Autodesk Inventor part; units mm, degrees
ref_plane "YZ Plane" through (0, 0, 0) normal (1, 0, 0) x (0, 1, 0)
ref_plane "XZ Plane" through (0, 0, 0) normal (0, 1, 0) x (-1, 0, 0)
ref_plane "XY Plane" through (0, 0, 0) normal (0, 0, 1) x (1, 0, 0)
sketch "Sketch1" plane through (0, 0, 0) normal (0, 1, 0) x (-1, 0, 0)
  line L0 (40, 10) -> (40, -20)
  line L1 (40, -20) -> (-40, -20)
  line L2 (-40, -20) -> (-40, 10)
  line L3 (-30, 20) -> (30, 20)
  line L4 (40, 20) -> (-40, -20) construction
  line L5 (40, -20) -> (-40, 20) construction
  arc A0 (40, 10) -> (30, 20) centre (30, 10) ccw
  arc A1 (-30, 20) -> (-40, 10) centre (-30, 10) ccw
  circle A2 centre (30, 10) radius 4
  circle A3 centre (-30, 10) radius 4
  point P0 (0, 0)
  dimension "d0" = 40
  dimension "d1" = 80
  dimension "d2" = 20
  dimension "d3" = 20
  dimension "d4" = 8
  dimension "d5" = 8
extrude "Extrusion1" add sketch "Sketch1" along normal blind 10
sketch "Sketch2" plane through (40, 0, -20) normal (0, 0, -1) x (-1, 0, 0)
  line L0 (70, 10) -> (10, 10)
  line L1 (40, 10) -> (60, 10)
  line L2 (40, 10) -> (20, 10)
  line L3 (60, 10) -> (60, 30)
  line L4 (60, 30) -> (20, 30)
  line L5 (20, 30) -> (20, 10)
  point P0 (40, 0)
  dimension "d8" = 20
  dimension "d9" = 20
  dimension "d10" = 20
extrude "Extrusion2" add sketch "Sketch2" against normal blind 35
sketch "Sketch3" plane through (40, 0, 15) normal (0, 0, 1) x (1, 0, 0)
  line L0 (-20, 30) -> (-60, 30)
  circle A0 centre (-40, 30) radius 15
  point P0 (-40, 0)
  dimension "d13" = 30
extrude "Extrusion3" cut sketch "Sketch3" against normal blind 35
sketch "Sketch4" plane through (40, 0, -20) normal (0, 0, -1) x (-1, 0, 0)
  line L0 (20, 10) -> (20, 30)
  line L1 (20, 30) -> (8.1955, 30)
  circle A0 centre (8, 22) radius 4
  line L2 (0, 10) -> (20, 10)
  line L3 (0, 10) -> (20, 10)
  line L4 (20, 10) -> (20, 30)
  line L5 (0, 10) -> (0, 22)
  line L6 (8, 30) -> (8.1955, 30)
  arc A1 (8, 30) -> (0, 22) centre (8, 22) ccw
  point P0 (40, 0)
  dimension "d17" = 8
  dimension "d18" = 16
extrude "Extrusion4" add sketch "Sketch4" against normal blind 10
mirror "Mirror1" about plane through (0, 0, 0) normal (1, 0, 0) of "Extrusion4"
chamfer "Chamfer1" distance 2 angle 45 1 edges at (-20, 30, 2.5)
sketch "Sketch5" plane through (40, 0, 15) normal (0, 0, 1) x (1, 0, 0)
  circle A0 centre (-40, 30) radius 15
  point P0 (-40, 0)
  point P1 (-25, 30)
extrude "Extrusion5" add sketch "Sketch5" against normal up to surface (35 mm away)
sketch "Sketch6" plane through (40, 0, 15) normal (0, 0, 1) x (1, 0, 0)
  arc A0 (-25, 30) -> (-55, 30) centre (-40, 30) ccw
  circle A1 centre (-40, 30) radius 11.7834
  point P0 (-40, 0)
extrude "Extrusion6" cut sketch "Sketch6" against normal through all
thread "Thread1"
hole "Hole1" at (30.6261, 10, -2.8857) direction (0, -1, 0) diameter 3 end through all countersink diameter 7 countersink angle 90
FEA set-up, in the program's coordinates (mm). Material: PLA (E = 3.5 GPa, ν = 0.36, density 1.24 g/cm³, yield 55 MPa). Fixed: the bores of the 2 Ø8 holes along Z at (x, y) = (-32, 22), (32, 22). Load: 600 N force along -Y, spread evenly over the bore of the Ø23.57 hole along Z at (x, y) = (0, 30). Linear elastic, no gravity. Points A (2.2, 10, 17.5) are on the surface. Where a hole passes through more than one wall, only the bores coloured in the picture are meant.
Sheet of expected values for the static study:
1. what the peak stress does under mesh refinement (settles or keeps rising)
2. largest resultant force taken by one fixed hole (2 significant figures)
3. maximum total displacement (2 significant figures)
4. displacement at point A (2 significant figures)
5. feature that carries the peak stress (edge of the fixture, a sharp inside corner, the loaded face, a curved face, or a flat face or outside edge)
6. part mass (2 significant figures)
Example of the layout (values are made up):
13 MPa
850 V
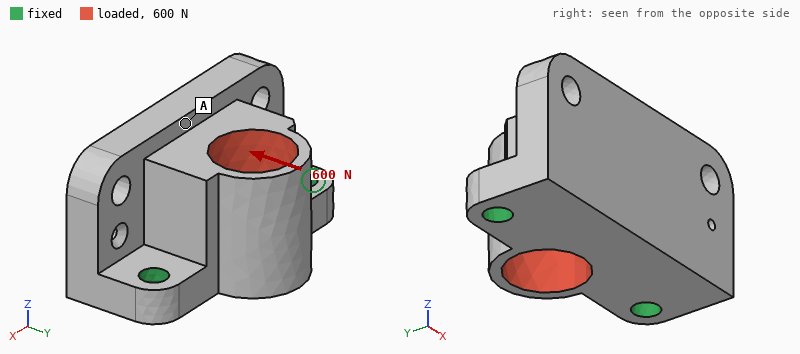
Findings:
keeps rising
340 N
0.20 mm
0.17 mm
edge of the fixture
77 g
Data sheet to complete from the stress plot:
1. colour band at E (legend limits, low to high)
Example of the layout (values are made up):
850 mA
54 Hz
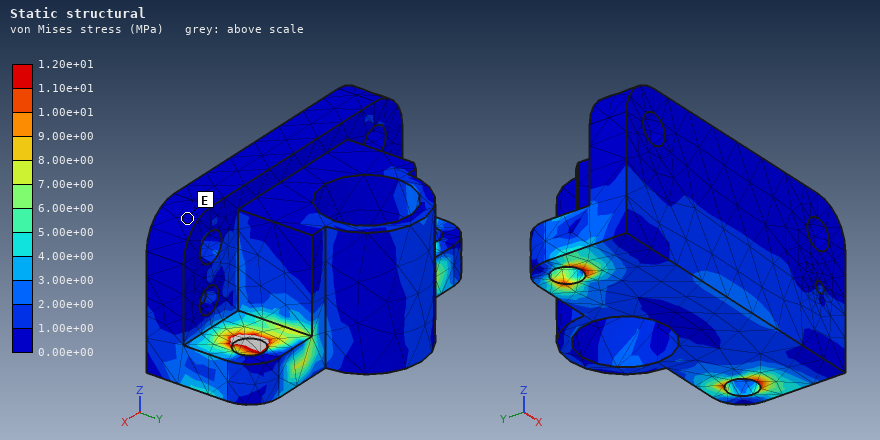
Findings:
0.00e+00 to 1.00e+00 MPa
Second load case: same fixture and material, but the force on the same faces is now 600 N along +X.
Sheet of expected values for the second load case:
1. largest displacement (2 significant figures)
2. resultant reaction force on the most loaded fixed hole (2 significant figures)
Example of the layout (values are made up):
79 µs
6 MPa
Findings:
90 µm
340 N
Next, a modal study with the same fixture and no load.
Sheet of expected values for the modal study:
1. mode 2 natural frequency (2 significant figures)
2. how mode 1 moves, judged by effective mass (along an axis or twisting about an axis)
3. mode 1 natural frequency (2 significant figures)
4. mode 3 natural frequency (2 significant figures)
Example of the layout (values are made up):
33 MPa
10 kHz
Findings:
3100 Hz
along Y
1200 Hz
3100 Hz
